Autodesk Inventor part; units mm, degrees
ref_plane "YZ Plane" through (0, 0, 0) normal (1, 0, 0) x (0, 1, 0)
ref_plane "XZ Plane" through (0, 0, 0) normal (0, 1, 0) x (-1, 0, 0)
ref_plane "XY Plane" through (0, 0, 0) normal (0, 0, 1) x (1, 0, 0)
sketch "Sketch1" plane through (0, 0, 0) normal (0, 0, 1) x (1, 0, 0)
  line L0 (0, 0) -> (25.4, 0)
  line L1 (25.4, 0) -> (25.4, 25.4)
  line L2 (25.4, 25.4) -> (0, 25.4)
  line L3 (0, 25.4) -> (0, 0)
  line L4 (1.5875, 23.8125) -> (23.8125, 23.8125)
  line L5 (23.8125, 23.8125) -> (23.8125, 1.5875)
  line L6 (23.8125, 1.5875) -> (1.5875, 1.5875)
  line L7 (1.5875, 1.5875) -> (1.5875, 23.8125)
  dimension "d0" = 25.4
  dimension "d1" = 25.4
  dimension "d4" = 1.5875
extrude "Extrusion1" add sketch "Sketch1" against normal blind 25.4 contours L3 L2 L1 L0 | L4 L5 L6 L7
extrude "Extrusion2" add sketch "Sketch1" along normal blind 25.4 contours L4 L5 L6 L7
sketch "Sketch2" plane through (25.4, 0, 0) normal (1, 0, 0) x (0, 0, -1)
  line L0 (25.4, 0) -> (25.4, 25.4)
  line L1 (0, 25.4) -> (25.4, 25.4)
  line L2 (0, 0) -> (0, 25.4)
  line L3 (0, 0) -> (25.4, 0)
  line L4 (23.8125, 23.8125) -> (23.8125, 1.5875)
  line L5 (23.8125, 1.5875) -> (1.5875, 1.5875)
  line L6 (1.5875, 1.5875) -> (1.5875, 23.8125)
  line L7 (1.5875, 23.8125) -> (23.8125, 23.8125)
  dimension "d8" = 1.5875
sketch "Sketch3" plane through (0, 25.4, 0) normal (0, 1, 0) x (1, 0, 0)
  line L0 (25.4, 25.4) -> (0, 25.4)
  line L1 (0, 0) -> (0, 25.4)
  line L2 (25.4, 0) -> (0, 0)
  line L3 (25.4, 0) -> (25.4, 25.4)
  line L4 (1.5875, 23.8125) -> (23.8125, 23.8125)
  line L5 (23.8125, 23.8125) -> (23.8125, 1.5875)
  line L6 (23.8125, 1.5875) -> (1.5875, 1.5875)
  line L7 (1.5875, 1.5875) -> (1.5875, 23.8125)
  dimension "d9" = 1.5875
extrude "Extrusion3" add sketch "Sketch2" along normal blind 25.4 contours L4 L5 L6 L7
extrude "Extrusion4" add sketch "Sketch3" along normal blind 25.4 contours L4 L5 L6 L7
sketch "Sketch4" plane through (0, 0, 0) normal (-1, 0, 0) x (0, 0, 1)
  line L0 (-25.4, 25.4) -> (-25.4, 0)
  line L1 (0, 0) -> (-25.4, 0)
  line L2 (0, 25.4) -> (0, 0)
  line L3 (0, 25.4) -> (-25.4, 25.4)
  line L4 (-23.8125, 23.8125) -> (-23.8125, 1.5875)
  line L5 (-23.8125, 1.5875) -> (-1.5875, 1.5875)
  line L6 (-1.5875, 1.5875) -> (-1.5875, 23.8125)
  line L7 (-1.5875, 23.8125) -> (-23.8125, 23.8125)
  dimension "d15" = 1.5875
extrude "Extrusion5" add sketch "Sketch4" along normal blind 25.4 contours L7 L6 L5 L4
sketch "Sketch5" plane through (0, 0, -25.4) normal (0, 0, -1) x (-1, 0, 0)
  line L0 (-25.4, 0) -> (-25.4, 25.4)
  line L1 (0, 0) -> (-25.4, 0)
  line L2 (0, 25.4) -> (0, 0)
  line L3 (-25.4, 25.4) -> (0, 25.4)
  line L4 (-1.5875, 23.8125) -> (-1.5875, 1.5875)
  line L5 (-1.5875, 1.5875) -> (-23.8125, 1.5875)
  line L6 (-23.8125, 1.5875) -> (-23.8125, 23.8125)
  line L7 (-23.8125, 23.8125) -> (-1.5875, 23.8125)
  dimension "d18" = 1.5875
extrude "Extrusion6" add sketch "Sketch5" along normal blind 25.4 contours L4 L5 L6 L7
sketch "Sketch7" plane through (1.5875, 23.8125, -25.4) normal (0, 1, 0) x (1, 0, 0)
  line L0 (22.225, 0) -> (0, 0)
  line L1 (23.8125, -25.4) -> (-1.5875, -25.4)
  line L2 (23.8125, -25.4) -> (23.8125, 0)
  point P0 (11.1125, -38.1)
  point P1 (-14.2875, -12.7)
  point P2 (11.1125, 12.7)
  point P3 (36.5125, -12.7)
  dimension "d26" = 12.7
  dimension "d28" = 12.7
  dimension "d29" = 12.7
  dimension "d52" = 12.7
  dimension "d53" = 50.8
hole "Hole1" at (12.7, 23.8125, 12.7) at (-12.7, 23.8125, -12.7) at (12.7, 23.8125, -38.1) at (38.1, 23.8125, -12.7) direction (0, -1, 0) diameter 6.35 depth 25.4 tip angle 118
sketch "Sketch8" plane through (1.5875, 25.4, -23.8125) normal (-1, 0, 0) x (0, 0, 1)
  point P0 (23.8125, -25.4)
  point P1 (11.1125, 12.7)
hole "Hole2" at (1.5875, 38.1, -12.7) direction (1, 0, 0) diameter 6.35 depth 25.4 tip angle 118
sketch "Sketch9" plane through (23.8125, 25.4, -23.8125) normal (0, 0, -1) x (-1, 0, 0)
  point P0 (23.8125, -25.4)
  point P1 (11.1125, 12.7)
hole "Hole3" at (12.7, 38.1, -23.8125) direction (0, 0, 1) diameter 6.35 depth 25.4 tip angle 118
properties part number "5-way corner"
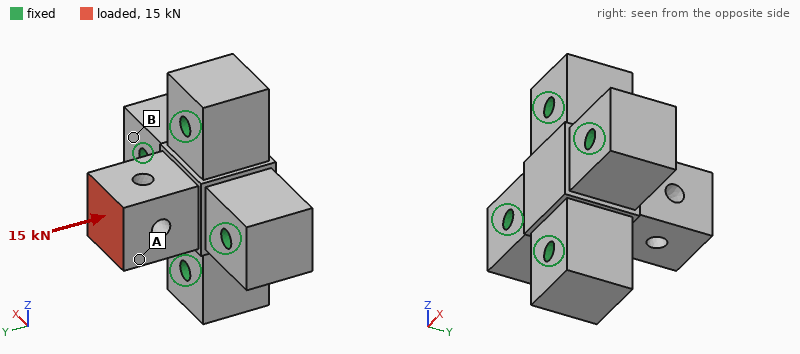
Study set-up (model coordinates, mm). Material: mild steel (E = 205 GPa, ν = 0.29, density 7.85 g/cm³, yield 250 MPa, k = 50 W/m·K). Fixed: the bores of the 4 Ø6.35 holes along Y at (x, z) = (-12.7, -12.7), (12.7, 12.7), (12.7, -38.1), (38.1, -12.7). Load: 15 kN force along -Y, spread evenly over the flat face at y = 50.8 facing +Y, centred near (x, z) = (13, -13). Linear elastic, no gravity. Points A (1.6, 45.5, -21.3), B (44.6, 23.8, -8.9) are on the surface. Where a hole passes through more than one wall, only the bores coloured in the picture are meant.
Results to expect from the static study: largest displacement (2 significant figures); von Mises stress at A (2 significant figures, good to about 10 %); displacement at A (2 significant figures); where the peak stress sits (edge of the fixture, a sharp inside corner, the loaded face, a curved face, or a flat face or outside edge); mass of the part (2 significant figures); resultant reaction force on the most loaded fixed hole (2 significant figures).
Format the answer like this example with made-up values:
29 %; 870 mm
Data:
8.5 µm; 37 MPa; 6.5 µm; a curved face; 590 g; 3.9 kN
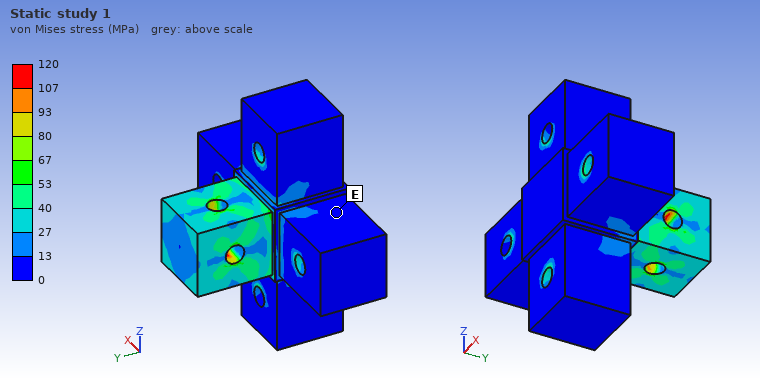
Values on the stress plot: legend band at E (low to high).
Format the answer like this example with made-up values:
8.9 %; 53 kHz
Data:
0 to 13 MPa
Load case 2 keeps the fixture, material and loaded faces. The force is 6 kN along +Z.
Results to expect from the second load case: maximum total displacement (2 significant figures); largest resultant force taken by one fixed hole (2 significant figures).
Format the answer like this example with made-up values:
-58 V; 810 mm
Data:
28 µm; 5.1 kN
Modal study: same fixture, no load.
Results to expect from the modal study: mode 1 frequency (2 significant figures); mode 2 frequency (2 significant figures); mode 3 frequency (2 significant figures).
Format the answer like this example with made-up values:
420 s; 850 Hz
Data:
13 kHz; 13 kHz; 23 kHz
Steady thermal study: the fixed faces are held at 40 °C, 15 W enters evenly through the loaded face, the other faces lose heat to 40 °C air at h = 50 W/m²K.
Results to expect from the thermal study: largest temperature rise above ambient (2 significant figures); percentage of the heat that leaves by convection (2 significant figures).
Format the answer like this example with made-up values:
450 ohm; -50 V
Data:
23 K; 16 %
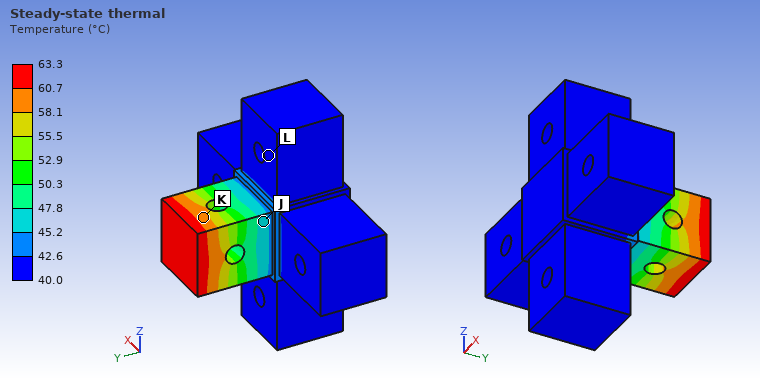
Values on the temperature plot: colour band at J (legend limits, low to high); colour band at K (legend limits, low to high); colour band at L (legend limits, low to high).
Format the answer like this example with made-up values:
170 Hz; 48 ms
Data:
45.2 to 47.8 °C; 58.1 to 60.7 °C; 40.0 to 42.6 °C
